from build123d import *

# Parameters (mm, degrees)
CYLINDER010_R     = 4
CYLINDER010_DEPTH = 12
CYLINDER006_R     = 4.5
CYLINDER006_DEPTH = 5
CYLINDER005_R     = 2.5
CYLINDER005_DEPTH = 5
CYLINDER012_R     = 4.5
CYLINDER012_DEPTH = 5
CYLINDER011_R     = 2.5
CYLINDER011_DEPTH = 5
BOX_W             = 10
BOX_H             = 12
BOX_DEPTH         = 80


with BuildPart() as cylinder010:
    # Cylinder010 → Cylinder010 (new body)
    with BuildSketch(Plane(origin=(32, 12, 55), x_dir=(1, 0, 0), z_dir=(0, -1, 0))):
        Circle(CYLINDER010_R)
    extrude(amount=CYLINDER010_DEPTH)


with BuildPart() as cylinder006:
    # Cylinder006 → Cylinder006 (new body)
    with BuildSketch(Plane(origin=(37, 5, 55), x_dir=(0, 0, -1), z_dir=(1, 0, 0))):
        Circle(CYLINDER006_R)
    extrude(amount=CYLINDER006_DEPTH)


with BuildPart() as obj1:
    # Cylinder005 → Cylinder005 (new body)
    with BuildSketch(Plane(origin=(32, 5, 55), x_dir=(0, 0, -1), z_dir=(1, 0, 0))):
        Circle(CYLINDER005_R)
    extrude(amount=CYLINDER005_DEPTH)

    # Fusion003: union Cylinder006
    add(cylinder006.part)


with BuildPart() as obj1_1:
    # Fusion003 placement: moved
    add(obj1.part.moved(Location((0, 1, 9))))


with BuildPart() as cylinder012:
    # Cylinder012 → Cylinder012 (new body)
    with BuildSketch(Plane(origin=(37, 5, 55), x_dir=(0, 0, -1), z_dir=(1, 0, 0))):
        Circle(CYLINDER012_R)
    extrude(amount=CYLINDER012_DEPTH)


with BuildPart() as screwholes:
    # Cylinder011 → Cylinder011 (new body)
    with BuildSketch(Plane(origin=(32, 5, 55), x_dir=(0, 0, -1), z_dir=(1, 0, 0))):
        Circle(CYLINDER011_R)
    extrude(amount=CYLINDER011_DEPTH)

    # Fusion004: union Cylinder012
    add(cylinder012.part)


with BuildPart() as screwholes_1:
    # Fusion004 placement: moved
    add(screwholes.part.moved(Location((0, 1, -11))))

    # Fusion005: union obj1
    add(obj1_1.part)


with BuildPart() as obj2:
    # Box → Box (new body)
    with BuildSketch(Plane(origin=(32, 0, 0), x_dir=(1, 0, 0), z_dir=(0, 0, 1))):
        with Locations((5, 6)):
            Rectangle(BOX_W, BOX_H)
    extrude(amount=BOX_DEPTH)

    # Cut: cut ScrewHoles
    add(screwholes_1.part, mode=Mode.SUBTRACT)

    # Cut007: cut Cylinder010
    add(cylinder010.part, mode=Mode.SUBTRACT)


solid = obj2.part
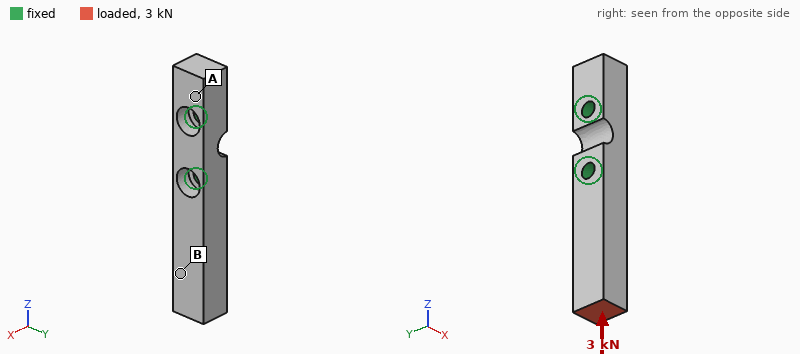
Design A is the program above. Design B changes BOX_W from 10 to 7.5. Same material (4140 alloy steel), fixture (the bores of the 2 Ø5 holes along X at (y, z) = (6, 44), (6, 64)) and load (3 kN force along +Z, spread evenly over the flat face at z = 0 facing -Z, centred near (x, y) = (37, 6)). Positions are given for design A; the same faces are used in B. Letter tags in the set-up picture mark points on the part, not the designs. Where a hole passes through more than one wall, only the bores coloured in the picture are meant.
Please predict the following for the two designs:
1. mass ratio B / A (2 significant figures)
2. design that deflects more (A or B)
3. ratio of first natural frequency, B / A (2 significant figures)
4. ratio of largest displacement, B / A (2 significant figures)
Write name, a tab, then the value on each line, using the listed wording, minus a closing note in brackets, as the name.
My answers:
mass ratio B / A	0.76
design that deflects more	B
ratio of first natural frequency, B / A	0.79
ratio of largest displacement, B / A	1.5
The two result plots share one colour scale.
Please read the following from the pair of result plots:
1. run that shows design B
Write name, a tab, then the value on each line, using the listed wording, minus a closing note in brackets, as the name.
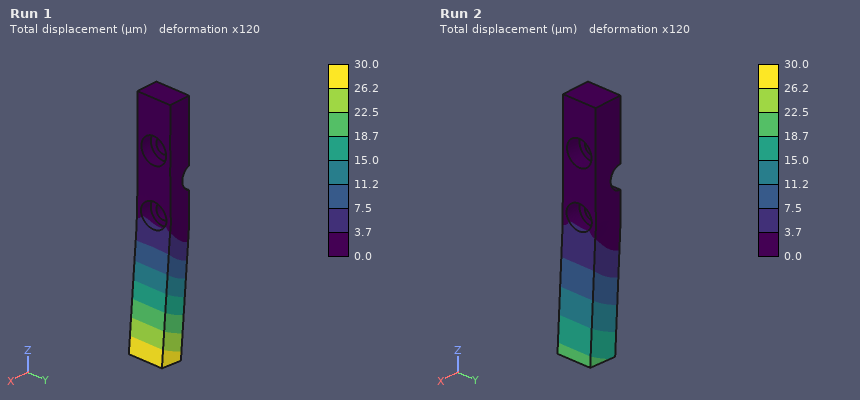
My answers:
run that shows design B	Run 1
